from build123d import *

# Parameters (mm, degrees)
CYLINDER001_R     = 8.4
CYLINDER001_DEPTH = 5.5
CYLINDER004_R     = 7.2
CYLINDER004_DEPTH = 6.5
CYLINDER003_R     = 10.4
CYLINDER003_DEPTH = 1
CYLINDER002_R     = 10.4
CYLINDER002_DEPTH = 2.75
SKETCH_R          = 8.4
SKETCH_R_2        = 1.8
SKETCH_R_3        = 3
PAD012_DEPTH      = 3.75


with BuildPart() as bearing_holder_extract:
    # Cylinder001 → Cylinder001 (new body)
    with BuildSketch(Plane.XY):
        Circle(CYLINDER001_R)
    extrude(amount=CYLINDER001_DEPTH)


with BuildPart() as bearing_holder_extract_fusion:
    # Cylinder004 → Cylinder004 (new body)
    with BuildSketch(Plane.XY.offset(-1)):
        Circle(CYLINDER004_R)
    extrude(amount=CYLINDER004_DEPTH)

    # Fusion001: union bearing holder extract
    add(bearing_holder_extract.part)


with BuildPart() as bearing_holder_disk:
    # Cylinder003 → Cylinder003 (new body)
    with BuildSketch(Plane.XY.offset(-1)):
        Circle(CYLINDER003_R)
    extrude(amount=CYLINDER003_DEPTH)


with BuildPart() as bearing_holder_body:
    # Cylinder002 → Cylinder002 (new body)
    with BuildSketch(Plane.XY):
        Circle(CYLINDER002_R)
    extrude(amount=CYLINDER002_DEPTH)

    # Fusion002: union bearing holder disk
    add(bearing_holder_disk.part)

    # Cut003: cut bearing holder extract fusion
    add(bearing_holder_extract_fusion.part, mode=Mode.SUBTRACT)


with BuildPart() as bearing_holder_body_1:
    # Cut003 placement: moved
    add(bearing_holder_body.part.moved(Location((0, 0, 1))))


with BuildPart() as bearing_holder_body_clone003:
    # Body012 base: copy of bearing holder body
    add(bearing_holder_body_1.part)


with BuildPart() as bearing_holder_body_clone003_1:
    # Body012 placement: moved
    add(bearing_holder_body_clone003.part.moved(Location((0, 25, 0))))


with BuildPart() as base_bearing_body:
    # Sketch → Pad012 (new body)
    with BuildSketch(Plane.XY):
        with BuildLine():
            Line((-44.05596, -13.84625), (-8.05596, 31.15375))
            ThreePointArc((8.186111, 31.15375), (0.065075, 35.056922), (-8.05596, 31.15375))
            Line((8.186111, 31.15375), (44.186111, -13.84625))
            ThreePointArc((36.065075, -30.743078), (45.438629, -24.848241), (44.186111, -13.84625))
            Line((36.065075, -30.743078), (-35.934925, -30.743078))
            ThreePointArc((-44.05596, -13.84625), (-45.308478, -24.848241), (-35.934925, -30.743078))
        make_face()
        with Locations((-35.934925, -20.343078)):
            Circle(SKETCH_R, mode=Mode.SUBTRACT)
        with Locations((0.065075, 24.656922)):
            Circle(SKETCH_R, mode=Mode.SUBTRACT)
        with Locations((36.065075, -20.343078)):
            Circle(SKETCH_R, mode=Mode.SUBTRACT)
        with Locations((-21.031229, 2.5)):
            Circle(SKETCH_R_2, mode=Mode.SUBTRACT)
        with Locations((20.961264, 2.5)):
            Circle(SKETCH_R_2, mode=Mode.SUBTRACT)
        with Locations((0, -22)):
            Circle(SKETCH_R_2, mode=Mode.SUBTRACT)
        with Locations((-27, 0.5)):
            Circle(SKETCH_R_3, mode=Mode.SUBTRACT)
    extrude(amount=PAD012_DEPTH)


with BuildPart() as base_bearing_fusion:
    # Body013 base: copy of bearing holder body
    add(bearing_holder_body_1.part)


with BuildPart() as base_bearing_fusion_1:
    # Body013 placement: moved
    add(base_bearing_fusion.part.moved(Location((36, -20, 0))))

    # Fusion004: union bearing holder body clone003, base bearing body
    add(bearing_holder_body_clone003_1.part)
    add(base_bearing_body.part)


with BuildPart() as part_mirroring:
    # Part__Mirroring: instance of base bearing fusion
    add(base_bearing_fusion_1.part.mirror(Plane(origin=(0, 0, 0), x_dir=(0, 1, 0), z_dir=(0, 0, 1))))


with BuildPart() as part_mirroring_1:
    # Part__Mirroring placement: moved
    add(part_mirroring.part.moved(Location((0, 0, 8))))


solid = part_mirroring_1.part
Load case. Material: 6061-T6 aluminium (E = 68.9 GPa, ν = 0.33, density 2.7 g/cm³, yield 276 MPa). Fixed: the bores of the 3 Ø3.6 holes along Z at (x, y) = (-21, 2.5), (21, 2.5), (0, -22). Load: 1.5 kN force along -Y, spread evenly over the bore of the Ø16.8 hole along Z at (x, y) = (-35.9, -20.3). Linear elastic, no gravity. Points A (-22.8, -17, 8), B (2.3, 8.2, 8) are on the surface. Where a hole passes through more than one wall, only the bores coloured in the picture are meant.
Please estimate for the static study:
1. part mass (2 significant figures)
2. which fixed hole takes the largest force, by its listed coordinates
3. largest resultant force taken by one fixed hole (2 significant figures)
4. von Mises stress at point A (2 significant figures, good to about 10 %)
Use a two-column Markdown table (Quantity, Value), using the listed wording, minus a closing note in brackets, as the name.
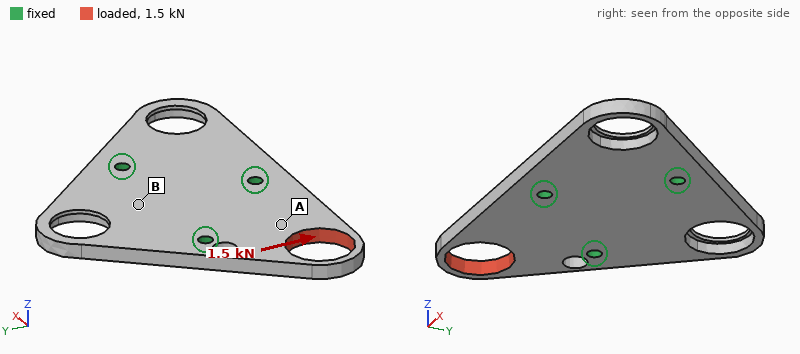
| Quantity | Value |
|---|---|
| part mass | 33 g |
| which fixed hole takes the largest force, by its listed coordinates | (-21, 2.5) |
| largest resultant force taken by one fixed hole | 1.6 kN |
| von Mises stress at point A | 40 MPa |
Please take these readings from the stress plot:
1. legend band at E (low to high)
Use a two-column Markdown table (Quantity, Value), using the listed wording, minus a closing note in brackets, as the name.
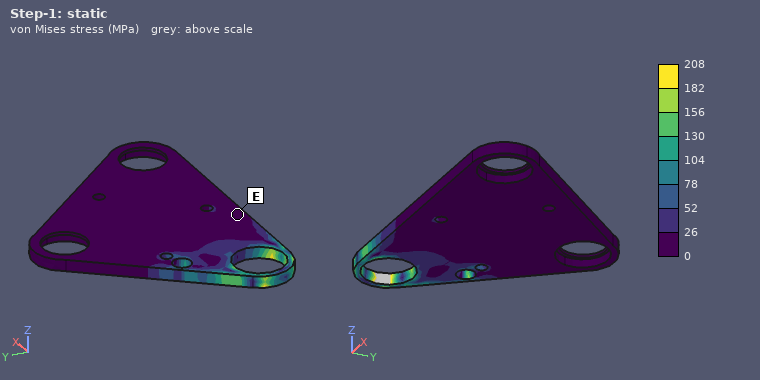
| Quantity | Value |
|---|---|
| legend band at E | 0 to 26 MPa |
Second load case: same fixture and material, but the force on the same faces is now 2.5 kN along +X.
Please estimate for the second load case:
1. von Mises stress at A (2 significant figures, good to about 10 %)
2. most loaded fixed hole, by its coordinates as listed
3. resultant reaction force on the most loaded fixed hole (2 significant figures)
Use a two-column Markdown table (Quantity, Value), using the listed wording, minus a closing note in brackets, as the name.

| Quantity | Value |
|---|---|
| von Mises stress at A | 27 MPa |
| most loaded fixed hole, by its coordinates as listed | (0, -22) |
| resultant reaction force on the most loaded fixed hole | 1.8 kN |
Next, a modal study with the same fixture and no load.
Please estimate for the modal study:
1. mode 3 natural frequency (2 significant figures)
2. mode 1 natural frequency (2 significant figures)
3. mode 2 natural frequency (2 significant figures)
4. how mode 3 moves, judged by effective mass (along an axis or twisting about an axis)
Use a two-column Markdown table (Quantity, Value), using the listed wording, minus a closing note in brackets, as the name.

| Quantity | Value |
|---|---|
| mode 3 natural frequency | 4500 Hz |
| mode 1 natural frequency | 3800 Hz |
| mode 2 natural frequency | 3900 Hz |
| how mode 3 moves, judged by effective mass | along Z |
